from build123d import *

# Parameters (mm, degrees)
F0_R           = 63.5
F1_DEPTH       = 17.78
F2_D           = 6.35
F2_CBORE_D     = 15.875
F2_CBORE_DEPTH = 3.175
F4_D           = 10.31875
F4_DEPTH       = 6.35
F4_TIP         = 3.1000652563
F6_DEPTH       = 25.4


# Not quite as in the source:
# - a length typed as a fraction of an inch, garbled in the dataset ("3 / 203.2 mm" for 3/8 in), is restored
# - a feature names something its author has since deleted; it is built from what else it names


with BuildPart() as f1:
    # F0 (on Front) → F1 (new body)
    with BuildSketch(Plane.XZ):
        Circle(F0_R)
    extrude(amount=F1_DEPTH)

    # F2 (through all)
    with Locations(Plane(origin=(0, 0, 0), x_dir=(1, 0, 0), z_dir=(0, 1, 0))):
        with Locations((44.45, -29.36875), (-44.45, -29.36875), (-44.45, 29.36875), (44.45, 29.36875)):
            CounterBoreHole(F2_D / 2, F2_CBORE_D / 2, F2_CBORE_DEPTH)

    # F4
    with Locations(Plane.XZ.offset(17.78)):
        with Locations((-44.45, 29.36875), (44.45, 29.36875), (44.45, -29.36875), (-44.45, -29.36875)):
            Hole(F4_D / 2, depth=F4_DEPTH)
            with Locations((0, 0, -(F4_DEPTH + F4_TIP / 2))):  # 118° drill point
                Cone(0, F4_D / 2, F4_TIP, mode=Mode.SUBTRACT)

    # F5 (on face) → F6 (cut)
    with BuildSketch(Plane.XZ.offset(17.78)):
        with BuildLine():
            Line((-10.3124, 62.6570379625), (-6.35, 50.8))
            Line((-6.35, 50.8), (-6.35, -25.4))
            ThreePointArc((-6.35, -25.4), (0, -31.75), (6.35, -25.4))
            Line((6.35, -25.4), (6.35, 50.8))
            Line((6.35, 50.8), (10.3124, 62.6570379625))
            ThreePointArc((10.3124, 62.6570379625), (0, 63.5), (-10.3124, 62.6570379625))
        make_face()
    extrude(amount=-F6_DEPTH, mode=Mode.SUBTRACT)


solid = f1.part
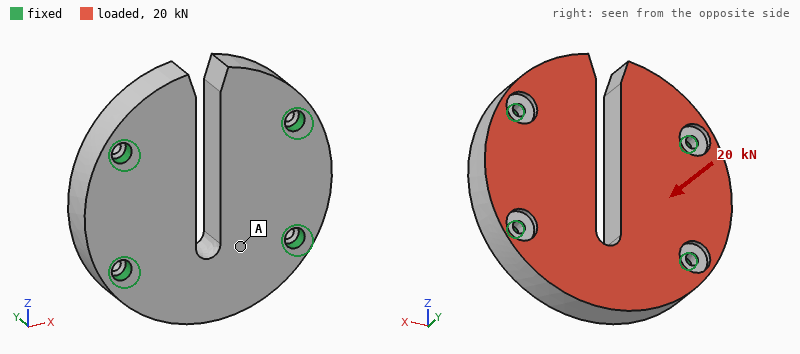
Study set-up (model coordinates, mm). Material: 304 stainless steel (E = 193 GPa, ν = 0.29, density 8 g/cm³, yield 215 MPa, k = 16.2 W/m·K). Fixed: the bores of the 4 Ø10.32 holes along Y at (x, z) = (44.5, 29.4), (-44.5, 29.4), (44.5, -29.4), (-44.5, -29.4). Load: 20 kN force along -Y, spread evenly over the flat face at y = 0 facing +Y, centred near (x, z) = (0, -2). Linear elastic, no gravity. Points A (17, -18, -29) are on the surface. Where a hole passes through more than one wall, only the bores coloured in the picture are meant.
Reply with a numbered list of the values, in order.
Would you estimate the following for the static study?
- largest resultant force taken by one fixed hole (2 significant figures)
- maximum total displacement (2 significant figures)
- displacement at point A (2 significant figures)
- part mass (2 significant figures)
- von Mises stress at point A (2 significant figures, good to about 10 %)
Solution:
1. 5.8 kN
2. 24 µm
3. 11 µm
4. 1.6 kg
5. 15 MPa
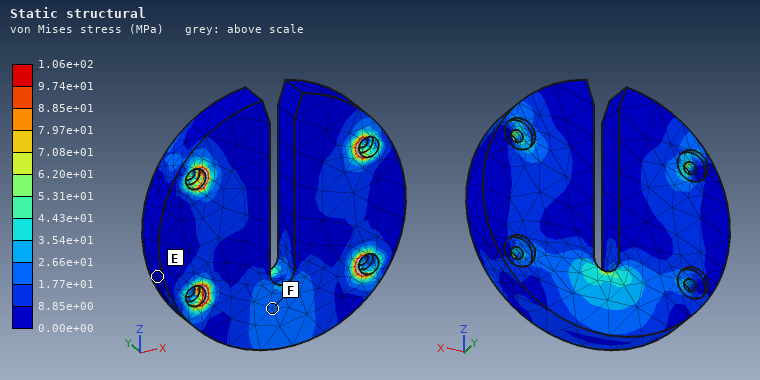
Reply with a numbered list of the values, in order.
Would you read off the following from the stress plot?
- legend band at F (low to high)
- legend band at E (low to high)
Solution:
1. 1.77e+01 to 2.66e+01 MPa
2. 0.00e+00 to 8.85e+00 MPa
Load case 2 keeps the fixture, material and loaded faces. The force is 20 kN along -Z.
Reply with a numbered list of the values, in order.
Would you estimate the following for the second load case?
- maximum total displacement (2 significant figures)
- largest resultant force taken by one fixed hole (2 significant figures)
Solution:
1. 10 µm
2. 5.6 kN
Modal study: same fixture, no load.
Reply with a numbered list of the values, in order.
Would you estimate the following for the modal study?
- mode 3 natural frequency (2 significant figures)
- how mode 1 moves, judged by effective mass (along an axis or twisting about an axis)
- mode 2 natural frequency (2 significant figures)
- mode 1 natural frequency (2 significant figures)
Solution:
1. 6000 Hz
2. along Y
3. 5100 Hz
4. 4700 Hz
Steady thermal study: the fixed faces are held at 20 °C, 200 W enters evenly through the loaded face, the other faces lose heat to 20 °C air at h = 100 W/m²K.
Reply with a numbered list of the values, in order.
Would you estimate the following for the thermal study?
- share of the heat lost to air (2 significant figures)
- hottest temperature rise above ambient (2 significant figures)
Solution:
1. 44 %
2. 68 K
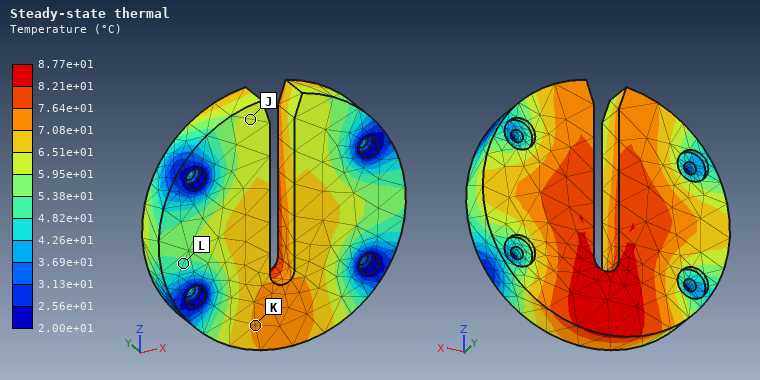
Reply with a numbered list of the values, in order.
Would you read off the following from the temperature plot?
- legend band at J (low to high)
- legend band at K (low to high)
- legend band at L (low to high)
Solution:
1. 5.95e+01 to 6.51e+01 °C
2. 7.08e+01 to 7.64e+01 °C
3. 4.82e+01 to 5.38e+01 °C
